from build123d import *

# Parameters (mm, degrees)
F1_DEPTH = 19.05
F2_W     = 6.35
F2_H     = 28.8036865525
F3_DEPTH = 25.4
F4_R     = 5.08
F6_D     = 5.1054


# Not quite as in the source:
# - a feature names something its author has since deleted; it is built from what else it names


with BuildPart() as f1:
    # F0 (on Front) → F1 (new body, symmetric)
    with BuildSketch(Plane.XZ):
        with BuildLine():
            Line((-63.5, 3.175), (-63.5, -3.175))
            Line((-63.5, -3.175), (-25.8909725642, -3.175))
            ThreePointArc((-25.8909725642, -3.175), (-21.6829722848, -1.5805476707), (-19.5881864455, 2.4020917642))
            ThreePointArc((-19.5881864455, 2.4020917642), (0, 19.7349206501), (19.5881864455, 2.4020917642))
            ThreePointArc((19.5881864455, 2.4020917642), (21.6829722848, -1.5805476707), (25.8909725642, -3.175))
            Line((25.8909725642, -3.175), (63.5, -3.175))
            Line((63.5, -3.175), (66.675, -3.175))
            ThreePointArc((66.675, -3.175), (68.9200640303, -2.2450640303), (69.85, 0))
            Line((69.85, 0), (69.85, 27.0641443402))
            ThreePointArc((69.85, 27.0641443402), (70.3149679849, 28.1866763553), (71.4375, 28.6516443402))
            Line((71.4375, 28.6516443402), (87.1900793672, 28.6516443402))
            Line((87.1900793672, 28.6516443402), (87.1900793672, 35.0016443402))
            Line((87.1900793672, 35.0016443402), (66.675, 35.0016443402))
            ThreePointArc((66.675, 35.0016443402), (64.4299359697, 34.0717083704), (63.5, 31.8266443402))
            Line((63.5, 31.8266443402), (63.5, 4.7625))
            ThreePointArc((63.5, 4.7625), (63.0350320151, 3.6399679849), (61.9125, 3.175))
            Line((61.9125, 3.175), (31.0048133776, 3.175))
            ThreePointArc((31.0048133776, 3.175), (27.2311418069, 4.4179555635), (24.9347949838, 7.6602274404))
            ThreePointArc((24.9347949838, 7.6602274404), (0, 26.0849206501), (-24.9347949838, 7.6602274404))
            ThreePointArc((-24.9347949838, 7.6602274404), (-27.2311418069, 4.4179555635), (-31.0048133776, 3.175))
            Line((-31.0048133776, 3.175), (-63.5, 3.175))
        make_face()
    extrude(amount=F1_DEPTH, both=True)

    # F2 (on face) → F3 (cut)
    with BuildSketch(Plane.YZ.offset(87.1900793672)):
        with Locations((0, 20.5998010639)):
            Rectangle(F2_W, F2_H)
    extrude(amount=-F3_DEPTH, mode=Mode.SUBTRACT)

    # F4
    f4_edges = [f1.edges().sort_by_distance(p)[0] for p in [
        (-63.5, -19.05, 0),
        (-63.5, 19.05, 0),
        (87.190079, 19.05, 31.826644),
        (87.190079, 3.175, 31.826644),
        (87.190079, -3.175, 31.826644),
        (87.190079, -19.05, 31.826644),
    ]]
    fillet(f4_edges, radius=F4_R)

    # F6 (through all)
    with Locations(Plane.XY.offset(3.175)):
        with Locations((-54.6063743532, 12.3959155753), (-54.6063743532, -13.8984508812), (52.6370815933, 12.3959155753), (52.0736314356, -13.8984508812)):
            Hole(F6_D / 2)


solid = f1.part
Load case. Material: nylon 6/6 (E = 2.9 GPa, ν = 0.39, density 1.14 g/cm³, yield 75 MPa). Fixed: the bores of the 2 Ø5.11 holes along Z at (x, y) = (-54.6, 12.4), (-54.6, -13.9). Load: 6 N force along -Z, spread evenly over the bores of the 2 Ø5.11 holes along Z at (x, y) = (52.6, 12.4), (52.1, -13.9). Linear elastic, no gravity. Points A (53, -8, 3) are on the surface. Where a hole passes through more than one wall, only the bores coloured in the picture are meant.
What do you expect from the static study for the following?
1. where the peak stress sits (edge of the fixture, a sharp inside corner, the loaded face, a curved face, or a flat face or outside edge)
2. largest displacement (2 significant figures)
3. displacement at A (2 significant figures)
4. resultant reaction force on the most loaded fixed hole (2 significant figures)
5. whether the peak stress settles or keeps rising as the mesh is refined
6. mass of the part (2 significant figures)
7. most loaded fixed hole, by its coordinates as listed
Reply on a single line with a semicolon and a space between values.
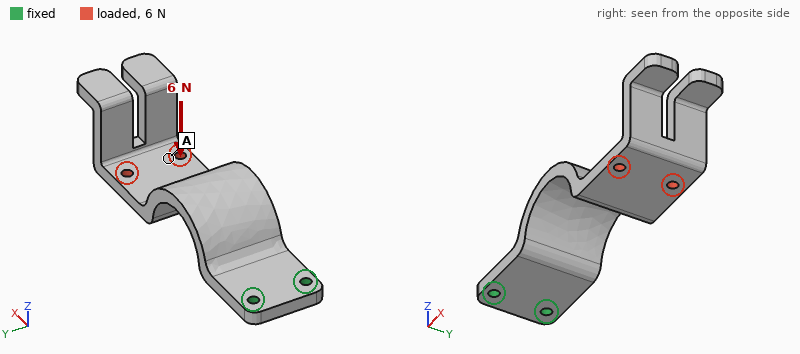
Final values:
edge of the fixture; 1.7 mm; 1.1 mm; 3.6 N; keeps rising; 54 g; (-54.6, 12.4)
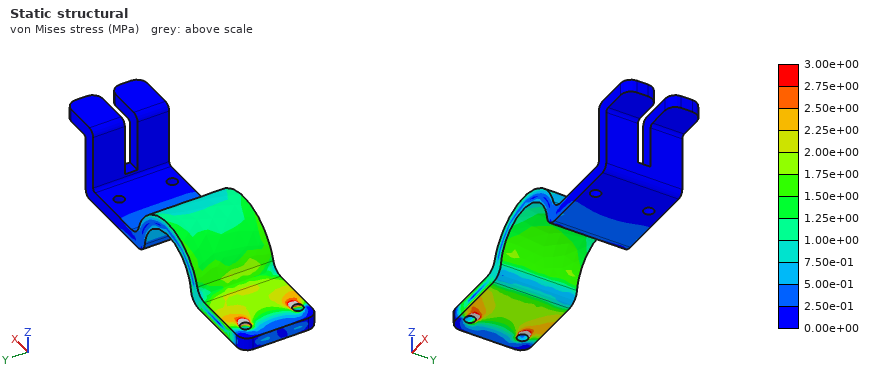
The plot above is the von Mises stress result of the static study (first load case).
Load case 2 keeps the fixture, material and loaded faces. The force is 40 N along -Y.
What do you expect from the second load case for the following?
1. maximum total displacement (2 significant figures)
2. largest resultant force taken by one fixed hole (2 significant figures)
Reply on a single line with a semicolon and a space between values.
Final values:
1.7 mm; 150 N
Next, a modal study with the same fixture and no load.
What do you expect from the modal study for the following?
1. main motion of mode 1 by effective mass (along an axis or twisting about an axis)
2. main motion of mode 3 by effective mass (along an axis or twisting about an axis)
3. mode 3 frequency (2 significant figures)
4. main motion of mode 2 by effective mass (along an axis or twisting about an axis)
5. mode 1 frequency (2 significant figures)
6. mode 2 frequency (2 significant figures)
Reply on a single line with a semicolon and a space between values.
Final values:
along Z; twisting about X; 320 Hz; along Y; 65 Hz; 170 Hz
